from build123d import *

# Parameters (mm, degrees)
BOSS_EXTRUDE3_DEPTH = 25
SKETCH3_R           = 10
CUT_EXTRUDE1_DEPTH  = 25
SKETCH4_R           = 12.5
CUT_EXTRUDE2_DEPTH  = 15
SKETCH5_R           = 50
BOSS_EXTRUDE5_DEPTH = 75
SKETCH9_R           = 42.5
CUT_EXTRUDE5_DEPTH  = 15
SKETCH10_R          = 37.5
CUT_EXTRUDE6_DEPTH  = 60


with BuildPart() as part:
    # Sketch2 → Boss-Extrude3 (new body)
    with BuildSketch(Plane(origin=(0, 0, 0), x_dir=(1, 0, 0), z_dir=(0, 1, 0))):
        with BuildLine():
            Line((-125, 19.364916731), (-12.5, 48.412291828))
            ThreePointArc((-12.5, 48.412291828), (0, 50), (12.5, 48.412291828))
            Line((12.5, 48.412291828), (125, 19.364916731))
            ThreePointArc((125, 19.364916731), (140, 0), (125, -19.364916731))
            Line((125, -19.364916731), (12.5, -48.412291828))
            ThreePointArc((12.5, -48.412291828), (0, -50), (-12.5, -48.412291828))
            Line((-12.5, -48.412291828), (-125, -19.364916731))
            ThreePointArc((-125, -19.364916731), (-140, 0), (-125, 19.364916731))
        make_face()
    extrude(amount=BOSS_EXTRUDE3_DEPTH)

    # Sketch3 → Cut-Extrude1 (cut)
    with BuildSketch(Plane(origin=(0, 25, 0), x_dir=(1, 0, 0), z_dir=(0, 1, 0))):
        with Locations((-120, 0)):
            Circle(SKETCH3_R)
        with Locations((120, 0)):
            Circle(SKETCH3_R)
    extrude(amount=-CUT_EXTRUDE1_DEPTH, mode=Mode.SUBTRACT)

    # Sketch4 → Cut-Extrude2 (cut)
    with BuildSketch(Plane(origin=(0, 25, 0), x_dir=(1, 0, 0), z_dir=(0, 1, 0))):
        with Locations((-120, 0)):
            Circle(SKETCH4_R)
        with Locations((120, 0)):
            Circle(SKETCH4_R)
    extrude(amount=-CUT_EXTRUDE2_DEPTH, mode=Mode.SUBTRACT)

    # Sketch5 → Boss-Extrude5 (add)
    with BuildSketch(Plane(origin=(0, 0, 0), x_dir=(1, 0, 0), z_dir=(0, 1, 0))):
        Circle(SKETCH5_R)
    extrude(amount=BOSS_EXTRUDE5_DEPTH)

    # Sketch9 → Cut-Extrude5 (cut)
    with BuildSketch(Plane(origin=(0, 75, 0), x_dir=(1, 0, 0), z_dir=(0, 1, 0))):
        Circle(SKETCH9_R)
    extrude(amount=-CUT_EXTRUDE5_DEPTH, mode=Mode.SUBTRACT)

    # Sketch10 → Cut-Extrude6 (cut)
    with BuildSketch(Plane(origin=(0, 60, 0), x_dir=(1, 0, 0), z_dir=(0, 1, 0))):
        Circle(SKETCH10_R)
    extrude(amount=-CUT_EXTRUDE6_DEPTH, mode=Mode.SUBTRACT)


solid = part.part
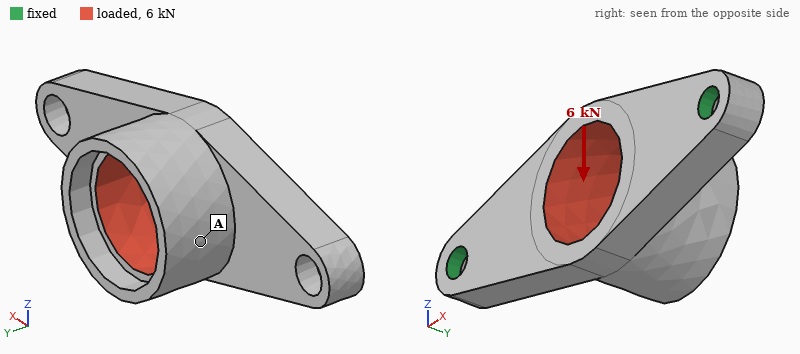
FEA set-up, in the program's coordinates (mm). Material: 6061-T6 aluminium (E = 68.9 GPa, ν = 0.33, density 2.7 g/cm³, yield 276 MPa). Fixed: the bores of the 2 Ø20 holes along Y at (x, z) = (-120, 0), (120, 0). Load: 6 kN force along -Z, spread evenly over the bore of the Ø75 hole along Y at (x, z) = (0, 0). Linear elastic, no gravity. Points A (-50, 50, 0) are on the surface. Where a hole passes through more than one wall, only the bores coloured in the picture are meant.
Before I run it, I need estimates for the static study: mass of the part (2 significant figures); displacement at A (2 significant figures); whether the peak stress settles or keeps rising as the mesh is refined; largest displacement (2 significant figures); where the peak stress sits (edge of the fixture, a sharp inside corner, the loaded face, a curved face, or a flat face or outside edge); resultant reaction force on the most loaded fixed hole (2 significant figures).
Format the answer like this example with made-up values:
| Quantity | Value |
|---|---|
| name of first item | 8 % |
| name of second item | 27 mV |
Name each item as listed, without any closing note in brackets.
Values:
| Quantity | Value |
|---|---|
| mass of the part | 1.3 kg |
| displacement at A | 0.069 mm |
| whether the peak stress settles or keeps rising as the mesh is refined | keeps rising |
| largest displacement | 0.12 mm |
| where the peak stress sits | edge of the fixture |
| resultant reaction force on the most loaded fixed hole | 3.0 kN |
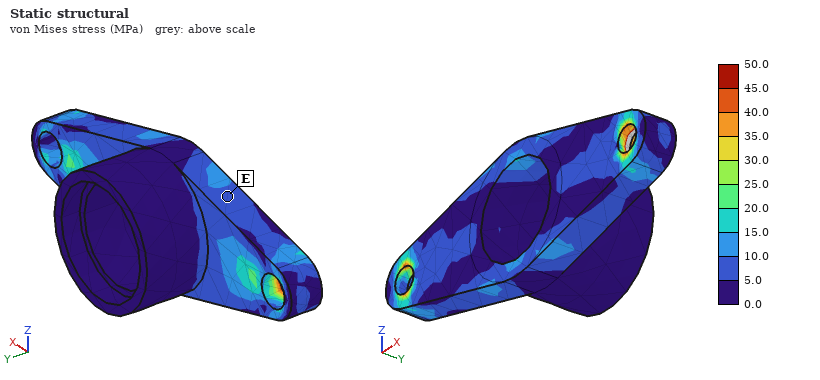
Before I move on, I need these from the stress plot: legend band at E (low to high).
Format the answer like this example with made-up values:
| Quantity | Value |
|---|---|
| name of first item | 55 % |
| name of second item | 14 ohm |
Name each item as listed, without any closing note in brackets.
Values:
| Quantity | Value |
|---|---|
| legend band at E | 5.0 to 10.0 MPa |
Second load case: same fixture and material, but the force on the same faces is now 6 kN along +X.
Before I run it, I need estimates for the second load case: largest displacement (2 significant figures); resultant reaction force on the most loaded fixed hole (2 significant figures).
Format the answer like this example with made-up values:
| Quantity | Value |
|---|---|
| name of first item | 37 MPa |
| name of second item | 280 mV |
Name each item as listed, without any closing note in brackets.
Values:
| Quantity | Value |
|---|---|
| largest displacement | 8.6 µm |
| resultant reaction force on the most loaded fixed hole | 3.1 kN |
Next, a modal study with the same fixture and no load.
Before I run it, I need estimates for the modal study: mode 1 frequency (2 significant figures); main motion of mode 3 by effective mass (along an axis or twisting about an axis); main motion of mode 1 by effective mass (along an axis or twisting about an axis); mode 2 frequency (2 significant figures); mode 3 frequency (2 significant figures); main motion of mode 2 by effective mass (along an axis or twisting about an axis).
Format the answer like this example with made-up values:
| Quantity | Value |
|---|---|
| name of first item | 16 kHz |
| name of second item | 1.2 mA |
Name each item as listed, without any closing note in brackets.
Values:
| Quantity | Value |
|---|---|
| mode 1 frequency | 1300 Hz |
| main motion of mode 3 by effective mass | along Z |
| main motion of mode 1 by effective mass | along Z |
| mode 2 frequency | 1500 Hz |
| mode 3 frequency | 3300 Hz |
| main motion of mode 2 by effective mass | along Y |
